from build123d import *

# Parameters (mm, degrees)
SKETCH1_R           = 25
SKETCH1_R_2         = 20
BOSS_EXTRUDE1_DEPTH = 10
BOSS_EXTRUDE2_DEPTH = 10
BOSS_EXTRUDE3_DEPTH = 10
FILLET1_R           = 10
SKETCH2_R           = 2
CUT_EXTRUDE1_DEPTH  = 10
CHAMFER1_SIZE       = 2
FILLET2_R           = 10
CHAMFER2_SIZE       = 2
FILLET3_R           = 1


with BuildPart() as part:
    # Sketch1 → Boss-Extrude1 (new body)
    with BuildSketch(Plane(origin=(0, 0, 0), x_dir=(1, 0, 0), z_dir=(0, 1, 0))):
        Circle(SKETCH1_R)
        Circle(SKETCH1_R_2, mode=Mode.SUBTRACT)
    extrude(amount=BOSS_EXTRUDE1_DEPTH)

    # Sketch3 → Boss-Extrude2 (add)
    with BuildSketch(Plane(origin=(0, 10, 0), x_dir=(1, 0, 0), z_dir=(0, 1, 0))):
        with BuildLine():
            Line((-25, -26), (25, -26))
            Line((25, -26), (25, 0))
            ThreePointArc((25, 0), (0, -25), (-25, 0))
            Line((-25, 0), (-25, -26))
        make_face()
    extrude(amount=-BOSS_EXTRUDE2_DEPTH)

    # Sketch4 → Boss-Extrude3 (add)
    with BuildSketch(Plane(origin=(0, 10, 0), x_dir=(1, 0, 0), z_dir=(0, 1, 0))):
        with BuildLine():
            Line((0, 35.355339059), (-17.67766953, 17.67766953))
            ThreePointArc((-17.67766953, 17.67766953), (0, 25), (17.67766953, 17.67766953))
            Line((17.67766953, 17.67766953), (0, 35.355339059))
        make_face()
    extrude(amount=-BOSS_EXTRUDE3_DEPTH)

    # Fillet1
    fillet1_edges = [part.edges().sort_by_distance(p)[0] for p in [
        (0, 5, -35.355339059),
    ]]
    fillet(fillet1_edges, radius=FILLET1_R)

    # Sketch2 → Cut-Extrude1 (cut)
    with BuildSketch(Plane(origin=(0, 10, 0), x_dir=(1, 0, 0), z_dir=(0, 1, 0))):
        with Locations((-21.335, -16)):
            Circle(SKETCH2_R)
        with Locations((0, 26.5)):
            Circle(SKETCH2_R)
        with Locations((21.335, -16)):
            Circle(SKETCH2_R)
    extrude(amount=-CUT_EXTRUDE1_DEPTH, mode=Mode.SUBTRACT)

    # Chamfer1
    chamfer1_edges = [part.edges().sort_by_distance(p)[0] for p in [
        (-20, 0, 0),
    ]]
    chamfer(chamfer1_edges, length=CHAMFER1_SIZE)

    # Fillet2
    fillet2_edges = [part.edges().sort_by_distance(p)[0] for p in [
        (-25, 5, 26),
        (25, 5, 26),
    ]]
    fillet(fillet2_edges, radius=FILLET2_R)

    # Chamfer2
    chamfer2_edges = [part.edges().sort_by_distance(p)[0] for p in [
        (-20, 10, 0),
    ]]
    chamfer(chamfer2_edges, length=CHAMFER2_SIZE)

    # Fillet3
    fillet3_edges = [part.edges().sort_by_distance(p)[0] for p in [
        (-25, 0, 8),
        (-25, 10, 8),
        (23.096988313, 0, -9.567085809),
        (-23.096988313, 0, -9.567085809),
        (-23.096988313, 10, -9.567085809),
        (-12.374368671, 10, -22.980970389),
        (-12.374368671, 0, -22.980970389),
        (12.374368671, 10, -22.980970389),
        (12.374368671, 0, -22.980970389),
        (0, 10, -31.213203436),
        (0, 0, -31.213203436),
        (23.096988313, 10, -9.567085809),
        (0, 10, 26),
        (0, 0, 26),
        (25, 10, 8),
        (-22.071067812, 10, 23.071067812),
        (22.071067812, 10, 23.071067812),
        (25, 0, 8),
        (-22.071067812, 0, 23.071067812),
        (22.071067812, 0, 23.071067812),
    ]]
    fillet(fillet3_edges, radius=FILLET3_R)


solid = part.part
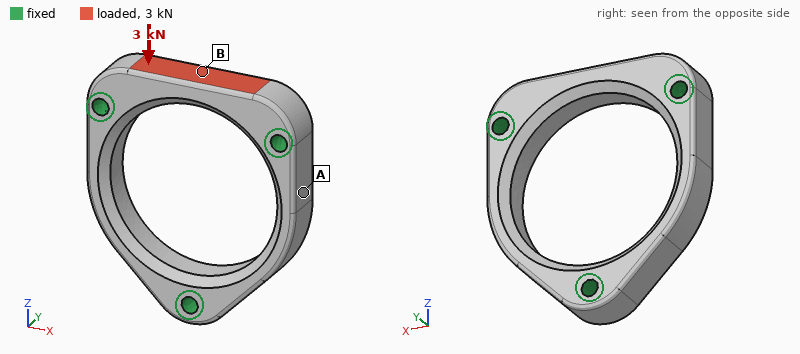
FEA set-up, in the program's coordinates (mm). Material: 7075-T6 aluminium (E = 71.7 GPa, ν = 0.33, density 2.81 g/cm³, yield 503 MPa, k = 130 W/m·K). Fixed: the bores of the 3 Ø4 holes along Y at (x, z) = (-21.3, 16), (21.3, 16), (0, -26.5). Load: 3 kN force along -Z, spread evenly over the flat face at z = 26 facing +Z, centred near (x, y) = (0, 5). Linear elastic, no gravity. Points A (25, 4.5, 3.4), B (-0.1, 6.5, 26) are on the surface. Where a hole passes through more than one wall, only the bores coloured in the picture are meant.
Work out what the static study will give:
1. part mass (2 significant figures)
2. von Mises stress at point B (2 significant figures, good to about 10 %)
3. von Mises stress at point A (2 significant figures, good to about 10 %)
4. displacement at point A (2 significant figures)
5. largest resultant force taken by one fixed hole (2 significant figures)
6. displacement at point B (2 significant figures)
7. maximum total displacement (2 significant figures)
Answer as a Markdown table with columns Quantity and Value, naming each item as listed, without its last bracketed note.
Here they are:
| Quantity | Value |
|---|---|
| part mass | 28 g |
| von Mises stress at point B | 65 MPa |
| von Mises stress at point A | 11 MPa |
| displacement at point A | 3.6 µm |
| largest resultant force taken by one fixed hole | 2.2 kN |
| displacement at point B | 22 µm |
| maximum total displacement | 23 µm |
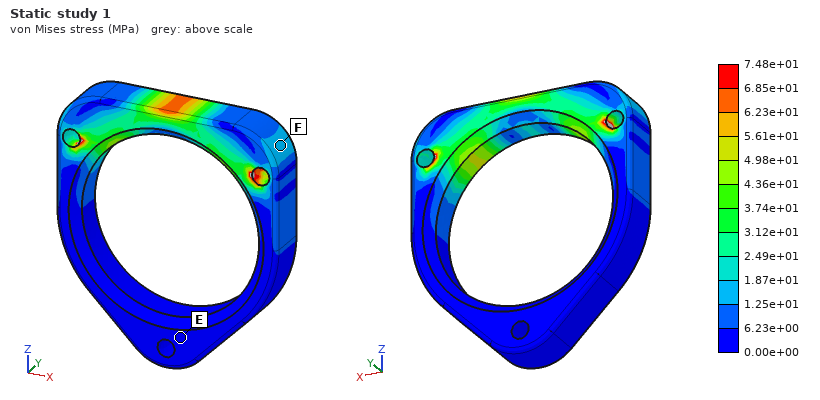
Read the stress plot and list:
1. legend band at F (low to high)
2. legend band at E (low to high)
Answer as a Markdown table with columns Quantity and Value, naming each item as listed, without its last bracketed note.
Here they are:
| Quantity | Value |
|---|---|
| legend band at F | 1.25e+01 to 1.87e+01 MPa |
| legend band at E | 0.00e+00 to 6.23e+00 MPa |
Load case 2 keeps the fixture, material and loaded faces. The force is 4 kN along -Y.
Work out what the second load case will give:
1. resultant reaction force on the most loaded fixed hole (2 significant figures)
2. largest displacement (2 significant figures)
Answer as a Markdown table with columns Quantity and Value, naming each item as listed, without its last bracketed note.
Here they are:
| Quantity | Value |
|---|---|
| resultant reaction force on the most loaded fixed hole | 2.0 kN |
| largest displacement | 68 µm |
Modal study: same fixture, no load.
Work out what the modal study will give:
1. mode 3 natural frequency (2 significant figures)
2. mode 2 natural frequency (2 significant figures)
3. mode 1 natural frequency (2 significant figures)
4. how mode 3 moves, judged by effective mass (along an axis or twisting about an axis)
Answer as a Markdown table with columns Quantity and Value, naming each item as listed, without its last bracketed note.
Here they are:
| Quantity | Value |
|---|---|
| mode 3 natural frequency | 22 kHz |
| mode 2 natural frequency | 17 kHz |
| mode 1 natural frequency | 16 kHz |
| how mode 3 moves, judged by effective mass | along Y |
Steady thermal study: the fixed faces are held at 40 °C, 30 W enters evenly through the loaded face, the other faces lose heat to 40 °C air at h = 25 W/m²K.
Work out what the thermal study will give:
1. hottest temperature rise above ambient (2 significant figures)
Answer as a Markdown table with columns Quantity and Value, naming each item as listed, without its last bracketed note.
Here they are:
| Quantity | Value |
|---|---|
| hottest temperature rise above ambient | 21 K |
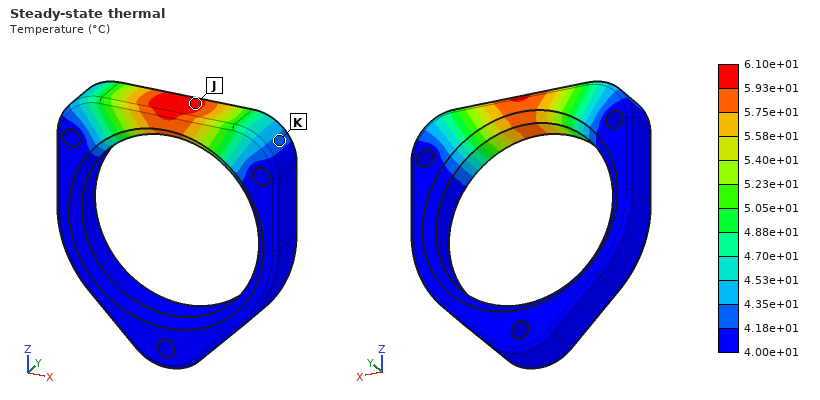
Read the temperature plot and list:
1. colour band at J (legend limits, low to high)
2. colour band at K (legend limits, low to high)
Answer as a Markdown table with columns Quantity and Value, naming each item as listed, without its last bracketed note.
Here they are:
| Quantity | Value |
|---|---|
| colour band at J | 5.93e+01 to 6.10e+01 °C |
| colour band at K | 4.18e+01 to 4.35e+01 °C |
